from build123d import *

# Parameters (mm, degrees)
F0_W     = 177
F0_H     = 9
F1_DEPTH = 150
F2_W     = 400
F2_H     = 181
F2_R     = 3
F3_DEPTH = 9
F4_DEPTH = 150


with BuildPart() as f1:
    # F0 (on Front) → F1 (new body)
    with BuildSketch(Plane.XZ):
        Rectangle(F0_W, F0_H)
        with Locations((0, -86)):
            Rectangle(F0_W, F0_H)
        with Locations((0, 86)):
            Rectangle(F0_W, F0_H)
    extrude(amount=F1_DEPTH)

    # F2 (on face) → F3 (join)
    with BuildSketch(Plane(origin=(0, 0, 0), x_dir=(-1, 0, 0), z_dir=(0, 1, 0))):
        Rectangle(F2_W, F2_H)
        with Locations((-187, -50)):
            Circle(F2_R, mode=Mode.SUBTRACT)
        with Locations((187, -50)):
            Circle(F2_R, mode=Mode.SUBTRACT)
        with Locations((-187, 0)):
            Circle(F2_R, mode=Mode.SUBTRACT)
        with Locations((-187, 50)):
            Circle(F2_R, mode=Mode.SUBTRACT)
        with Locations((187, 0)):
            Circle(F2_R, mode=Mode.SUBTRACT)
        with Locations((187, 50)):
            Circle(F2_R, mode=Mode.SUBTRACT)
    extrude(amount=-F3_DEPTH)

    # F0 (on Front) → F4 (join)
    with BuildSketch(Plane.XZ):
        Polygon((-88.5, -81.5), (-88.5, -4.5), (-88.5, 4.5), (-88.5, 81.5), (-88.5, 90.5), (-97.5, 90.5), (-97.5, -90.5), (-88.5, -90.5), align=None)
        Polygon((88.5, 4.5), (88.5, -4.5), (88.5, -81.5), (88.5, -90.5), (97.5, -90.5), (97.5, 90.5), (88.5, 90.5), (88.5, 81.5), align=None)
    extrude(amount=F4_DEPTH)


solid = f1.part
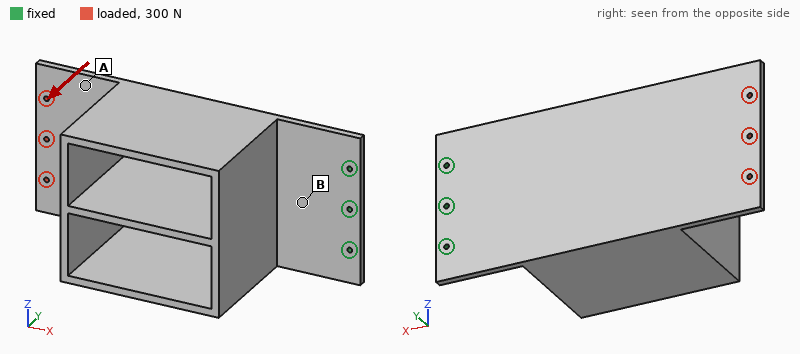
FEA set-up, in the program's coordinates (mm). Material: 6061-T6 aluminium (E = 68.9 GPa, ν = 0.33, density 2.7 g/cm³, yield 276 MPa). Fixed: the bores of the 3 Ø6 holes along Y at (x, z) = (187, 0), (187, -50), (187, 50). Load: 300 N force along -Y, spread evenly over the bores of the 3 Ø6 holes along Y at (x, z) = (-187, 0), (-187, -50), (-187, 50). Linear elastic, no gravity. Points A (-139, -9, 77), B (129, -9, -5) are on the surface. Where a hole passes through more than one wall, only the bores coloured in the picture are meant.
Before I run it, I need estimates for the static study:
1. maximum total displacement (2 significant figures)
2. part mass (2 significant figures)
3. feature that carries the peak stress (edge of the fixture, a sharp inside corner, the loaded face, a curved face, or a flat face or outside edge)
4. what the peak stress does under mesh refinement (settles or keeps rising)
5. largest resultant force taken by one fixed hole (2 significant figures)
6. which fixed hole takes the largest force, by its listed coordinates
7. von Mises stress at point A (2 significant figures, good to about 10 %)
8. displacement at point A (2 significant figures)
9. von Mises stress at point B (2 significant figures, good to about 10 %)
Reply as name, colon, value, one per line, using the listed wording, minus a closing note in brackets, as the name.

maximum total displacement: 4.5 mm
part mass: 4.8 kg
feature that carries the peak stress: edge of the fixture
what the peak stress does under mesh refinement: keeps rising
largest resultant force taken by one fixed hole: 260 N
which fixed hole takes the largest force, by its listed coordinates: (187, 0)
von Mises stress at point A: 5.9 MPa
displacement at point A: 3.6 mm
von Mises stress at point B: 35 MPa
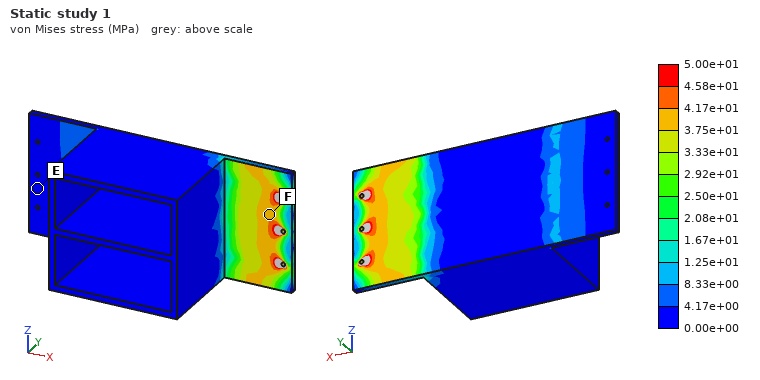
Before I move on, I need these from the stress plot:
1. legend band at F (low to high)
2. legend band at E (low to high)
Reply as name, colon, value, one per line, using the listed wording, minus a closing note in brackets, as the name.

legend band at F: 3.75e+01 to 4.17e+01 MPa
legend band at E: 0.00e+00 to 4.17e+00 MPa
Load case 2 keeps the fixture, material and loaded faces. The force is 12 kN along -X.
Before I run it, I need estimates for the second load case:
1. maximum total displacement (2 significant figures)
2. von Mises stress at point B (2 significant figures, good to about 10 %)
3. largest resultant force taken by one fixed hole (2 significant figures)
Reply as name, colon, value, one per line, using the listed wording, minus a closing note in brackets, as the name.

maximum total displacement: 96 µm
von Mises stress at point B: 8.4 MPa
largest resultant force taken by one fixed hole: 4.2 kN
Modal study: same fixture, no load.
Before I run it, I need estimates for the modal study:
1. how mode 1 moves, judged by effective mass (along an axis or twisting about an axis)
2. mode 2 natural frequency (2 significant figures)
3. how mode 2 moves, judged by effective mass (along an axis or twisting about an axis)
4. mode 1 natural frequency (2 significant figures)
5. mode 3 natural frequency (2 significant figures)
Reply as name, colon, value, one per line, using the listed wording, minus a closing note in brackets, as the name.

how mode 1 moves, judged by effective mass: along Y
mode 2 natural frequency: 130 Hz
how mode 2 moves, judged by effective mass: along Z
mode 1 natural frequency: 35 Hz
mode 3 natural frequency: 390 Hz
